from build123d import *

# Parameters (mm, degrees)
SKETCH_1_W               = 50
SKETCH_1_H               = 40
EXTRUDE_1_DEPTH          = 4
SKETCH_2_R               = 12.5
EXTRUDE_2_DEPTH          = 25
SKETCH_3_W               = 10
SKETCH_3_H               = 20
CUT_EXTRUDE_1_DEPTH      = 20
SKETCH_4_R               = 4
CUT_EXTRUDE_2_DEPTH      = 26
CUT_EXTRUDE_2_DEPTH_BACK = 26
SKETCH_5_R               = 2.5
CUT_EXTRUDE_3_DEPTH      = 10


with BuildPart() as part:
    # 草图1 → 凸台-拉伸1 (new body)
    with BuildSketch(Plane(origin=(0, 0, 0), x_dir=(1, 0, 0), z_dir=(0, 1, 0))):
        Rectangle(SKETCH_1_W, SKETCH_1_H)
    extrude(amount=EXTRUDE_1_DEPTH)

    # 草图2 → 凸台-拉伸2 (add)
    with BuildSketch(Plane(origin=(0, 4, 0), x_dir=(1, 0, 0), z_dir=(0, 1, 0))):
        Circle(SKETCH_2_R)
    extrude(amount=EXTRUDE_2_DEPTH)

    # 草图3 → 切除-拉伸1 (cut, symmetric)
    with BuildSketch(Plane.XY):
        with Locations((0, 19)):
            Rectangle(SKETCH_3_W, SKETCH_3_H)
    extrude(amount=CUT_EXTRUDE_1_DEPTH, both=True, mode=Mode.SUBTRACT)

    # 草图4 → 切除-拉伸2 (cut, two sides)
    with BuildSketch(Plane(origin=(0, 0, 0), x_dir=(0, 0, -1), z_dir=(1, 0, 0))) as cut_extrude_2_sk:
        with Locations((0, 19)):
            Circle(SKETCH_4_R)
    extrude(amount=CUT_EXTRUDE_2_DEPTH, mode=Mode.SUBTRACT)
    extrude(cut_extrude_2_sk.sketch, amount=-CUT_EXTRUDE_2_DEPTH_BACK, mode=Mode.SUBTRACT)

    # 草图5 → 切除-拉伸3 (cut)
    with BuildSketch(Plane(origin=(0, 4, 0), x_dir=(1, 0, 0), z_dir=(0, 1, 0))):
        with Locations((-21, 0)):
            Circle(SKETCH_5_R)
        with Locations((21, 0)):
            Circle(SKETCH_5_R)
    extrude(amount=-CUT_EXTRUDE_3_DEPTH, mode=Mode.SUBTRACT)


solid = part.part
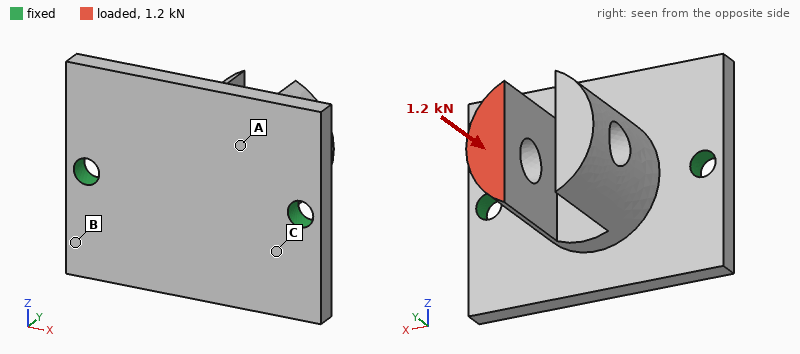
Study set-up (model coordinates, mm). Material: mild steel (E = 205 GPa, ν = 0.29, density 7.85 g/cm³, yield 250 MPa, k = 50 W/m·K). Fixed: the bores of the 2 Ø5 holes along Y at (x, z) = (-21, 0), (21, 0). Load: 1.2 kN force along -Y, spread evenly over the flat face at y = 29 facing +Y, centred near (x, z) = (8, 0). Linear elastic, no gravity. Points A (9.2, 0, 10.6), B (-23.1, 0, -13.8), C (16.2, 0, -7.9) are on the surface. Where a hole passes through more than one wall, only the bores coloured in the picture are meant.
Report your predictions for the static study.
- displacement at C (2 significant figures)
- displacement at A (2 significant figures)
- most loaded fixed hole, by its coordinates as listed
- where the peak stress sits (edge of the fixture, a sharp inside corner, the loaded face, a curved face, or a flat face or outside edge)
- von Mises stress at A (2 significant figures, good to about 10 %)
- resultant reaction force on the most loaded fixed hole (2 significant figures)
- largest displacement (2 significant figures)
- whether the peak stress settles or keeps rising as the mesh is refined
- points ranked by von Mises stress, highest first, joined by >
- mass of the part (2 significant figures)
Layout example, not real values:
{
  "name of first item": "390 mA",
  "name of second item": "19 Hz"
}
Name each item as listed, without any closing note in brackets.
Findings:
{
  "displacement at C": "3.1 µm",
  "displacement at A": "5.3 µm",
  "most loaded fixed hole, by its coordinates as listed": "(21, 0)",
  "where the peak stress sits": "edge of the fixture",
  "von Mises stress at A": "20 MPa",
  "resultant reaction force on the most loaded fixed hole": "930 N",
  "largest displacement": "8.2 µm",
  "whether the peak stress settles or keeps rising as the mesh is refined": "keeps rising",
  "points ranked by von Mises stress, highest first, joined by >": "A > C > B",
  "mass of the part": "110 g"
}
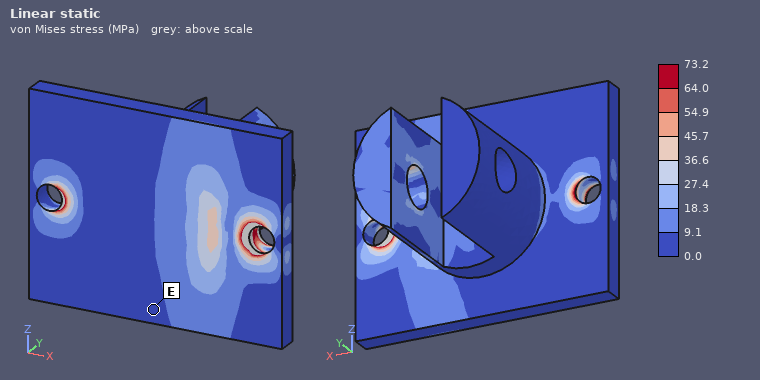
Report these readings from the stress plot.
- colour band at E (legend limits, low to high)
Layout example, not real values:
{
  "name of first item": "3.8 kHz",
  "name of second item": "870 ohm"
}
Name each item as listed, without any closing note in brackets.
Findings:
{
  "colour band at E": "0.0 to 9.1 MPa"
}
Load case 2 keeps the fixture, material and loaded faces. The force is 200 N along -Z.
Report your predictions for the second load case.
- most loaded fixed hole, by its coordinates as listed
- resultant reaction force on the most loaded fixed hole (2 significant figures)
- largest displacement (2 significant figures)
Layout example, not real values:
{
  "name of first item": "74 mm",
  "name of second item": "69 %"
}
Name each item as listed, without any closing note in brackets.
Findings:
{
  "most loaded fixed hole, by its coordinates as listed": "(21, 0)",
  "resultant reaction force on the most loaded fixed hole": "130 N",
  "largest displacement": "20 µm"
}
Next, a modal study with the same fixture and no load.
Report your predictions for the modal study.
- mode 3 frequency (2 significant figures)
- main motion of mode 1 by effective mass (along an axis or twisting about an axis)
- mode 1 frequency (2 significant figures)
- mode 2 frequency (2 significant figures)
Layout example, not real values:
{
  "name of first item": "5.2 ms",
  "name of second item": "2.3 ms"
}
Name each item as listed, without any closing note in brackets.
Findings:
{
  "mode 3 frequency": "7700 Hz",
  "main motion of mode 1 by effective mass": "along Z",
  "mode 1 frequency": "3500 Hz",
  "mode 2 frequency": "7500 Hz"
}
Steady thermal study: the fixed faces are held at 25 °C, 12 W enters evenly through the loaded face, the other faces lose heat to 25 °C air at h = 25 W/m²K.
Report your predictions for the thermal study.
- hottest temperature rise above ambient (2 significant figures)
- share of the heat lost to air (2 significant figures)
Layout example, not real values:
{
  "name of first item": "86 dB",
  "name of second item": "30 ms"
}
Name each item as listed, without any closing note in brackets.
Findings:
{
  "hottest temperature rise above ambient": "71 K",
  "share of the heat lost to air": "21 %"
}
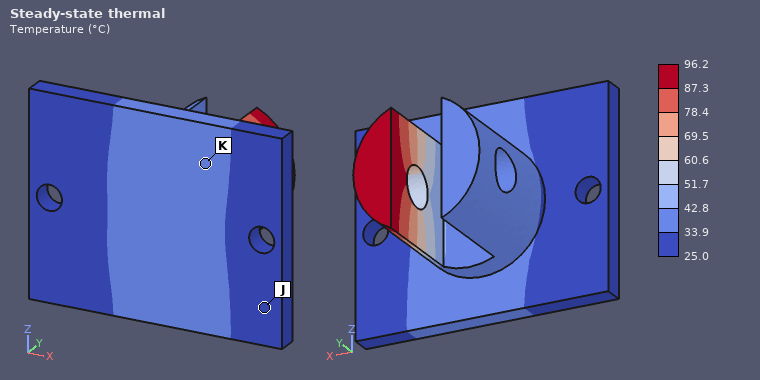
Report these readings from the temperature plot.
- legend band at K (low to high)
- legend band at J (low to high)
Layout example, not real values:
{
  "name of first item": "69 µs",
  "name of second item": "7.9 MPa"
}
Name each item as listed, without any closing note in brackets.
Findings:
{
  "legend band at K": "33.9 to 42.8 °C",
  "legend band at J": "25.0 to 33.9 °C"
}
